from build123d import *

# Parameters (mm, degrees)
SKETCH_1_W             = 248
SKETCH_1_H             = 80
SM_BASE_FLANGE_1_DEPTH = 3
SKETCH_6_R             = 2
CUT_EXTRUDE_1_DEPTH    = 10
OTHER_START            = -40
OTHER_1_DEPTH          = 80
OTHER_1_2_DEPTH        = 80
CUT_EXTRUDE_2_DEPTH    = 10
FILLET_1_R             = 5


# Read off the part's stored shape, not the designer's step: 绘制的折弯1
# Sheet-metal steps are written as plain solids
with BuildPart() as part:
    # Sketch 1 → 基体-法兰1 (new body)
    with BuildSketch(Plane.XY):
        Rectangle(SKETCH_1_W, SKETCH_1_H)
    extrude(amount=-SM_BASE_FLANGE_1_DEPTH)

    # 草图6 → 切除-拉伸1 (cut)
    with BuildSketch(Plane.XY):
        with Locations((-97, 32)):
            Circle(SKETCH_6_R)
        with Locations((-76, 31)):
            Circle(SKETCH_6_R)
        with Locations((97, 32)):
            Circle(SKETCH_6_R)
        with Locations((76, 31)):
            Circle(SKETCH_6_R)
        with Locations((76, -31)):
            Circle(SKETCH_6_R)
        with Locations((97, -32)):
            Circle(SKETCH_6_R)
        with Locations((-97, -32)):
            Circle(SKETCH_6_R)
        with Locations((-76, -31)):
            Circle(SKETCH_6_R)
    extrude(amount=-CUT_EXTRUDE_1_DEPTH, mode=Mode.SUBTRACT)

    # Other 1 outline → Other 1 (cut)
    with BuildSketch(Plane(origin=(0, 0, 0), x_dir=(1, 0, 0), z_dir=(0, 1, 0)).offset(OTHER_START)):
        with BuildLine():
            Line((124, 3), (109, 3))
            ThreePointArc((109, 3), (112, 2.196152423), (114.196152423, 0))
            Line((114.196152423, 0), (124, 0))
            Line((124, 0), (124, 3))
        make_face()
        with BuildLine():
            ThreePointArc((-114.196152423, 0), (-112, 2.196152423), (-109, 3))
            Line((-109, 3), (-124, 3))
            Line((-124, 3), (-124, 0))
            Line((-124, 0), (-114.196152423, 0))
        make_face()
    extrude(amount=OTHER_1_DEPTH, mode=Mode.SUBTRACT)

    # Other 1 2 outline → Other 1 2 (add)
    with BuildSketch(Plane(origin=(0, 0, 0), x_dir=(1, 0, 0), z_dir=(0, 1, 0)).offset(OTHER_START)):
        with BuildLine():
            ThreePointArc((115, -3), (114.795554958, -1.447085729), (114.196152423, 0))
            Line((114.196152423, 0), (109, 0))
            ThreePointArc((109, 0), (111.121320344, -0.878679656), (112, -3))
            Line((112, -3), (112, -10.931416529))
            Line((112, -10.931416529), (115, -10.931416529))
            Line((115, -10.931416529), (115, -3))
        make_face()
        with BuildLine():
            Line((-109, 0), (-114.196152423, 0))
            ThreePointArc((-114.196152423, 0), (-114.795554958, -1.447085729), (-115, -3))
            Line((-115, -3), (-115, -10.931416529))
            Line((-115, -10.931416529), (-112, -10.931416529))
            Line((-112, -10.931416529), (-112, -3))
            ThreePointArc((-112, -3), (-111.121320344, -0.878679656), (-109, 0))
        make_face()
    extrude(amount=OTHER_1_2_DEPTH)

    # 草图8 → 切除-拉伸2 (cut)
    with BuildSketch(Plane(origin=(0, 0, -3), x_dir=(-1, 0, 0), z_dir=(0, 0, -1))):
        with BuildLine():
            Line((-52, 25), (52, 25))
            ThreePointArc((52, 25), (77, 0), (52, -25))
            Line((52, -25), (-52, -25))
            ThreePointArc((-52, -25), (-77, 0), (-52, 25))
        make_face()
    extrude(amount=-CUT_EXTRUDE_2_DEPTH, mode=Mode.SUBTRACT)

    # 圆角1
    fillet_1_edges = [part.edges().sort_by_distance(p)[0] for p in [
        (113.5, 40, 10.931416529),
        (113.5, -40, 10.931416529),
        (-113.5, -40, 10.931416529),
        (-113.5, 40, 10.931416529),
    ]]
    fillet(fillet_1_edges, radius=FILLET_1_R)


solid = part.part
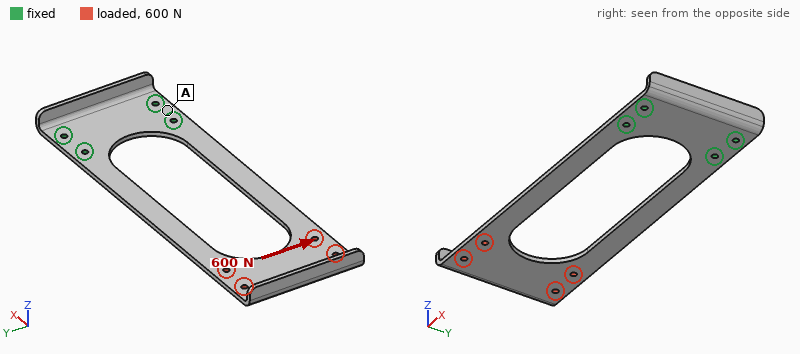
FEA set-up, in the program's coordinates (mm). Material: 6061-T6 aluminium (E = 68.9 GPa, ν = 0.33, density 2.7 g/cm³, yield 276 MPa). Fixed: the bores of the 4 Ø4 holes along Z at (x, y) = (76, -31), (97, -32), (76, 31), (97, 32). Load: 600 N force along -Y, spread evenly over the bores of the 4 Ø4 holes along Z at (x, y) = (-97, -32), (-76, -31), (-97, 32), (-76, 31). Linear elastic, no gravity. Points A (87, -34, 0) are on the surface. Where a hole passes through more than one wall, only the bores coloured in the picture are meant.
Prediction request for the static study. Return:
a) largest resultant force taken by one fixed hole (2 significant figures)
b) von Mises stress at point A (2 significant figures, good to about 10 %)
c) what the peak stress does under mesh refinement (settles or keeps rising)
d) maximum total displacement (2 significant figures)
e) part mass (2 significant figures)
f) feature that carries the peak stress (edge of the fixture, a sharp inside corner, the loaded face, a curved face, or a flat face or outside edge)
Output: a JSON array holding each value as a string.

["1.3 kN", "23 MPa", "keeps rising", "1.4 mm", "100 g", "edge of the fixture"]
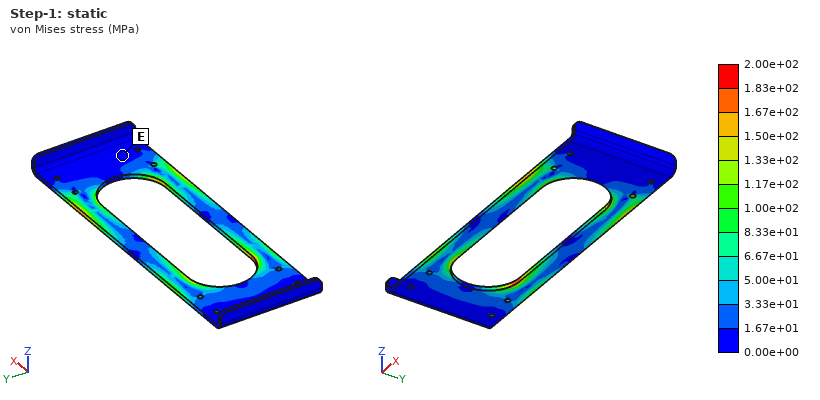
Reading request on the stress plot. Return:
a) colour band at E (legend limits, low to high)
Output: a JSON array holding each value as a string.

["0.00e+00 to 1.67e+01 MPa"]
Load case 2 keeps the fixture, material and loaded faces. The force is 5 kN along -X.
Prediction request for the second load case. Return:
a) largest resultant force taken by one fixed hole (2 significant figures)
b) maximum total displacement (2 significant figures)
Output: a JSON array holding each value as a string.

["2.1 kN", "0.13 mm"]
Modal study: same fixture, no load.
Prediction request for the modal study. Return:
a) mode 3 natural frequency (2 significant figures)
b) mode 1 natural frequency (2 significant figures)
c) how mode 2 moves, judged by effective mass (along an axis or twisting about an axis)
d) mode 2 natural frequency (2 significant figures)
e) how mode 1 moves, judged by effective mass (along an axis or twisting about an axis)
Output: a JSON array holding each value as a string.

["360 Hz", "44 Hz", "twisting about X", "210 Hz", "along Z"]
